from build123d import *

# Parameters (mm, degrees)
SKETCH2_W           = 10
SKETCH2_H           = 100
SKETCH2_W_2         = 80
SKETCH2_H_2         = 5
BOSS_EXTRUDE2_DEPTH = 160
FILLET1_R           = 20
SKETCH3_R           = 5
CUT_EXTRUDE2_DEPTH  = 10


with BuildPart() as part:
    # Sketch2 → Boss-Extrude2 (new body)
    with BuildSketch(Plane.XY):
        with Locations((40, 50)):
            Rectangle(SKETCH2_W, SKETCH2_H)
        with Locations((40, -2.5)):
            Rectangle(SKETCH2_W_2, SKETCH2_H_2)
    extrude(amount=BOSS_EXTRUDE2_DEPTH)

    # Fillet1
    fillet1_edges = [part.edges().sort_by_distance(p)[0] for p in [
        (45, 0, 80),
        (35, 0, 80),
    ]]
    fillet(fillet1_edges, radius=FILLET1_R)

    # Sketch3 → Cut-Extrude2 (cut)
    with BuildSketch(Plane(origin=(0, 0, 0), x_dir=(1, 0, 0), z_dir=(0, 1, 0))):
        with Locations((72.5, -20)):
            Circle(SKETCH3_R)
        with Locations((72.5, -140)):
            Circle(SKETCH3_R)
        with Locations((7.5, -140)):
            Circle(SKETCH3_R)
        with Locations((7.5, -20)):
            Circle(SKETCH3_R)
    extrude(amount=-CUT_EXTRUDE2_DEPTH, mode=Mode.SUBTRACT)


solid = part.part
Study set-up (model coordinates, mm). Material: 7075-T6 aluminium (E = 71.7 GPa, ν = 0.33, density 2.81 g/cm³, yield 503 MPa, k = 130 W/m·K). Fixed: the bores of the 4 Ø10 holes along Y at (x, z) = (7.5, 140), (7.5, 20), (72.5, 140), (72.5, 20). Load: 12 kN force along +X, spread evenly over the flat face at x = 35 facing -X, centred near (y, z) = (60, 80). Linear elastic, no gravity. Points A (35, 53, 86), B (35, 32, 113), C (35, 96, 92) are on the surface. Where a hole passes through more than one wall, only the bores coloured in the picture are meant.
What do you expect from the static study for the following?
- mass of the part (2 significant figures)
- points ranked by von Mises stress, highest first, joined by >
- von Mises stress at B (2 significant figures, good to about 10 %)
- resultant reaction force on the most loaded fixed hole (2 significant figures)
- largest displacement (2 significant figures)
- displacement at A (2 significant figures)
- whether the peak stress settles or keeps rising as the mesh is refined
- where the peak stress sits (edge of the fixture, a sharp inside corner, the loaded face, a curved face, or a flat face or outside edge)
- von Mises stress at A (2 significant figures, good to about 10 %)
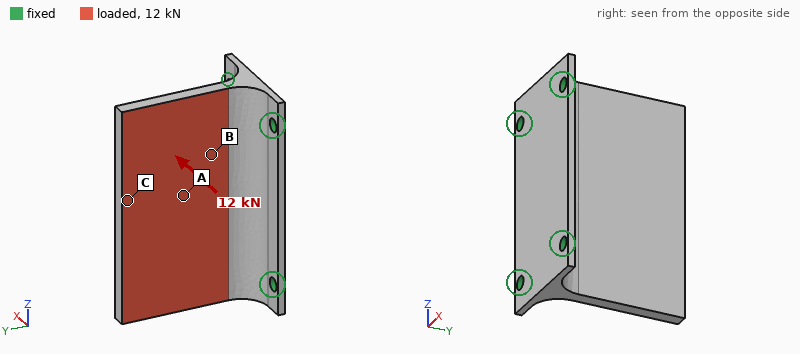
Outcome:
700 g
B > A > C
110 MPa
8.1 kN
1.9 mm
0.81 mm
keeps rising
edge of the fixture
57 MPa
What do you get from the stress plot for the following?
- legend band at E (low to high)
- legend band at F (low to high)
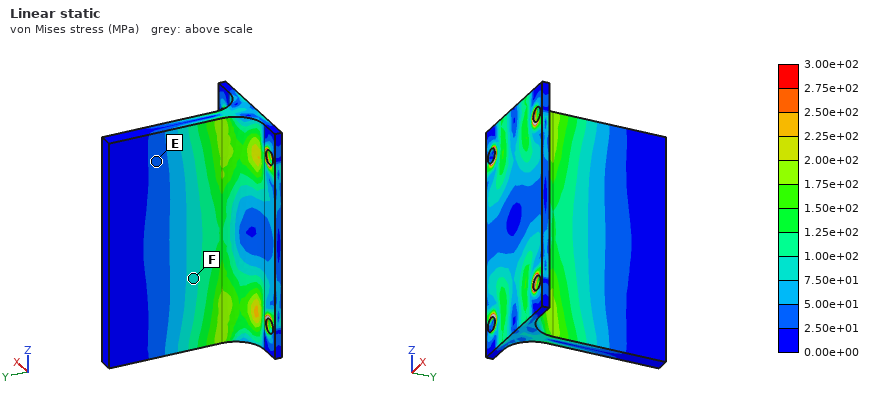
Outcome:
2.50e+01 to 5.00e+01 MPa
7.50e+01 to 1.00e+02 MPa
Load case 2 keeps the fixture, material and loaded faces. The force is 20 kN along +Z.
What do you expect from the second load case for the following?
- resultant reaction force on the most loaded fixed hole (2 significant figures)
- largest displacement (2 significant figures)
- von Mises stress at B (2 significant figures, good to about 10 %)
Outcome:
9.0 kN
0.30 mm
34 MPa
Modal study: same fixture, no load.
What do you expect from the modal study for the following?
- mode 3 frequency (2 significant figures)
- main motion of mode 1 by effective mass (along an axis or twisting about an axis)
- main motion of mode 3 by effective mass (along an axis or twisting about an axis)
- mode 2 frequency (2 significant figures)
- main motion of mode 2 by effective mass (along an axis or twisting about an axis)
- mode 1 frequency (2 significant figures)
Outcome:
2400 Hz
along X
along Z
1500 Hz
twisting about Y
830 Hz
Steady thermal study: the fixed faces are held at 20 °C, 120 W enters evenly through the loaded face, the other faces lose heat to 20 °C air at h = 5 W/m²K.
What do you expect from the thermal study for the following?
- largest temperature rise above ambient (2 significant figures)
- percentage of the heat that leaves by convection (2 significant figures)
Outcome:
53 K
5.3 %
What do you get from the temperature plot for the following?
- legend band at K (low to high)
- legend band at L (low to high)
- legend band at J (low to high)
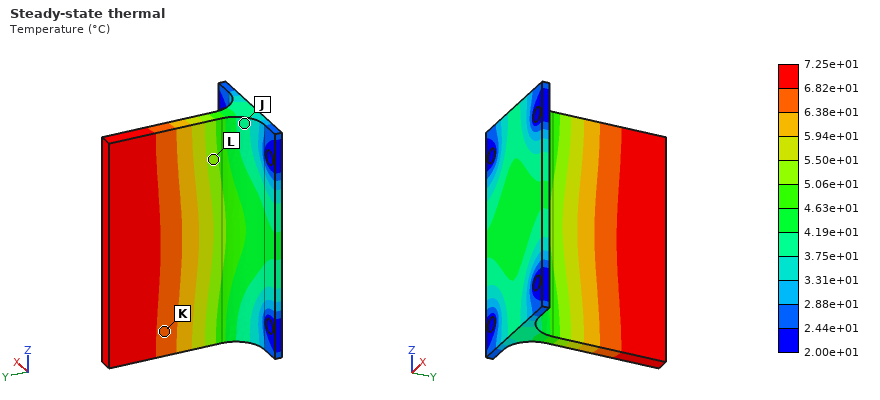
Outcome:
6.38e+01 to 6.82e+01 °C
5.06e+01 to 5.50e+01 °C
3.75e+01 to 4.19e+01 °C
